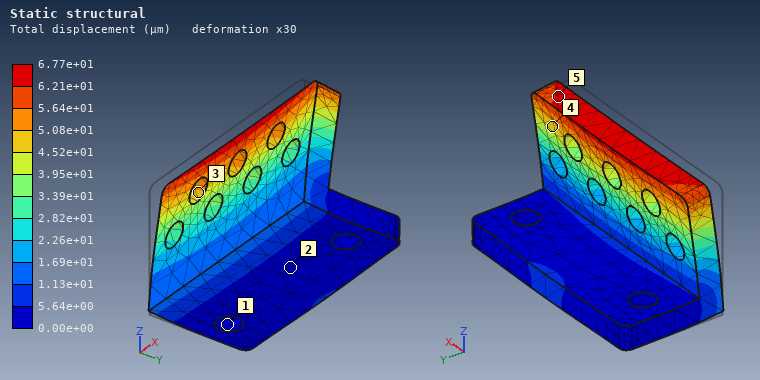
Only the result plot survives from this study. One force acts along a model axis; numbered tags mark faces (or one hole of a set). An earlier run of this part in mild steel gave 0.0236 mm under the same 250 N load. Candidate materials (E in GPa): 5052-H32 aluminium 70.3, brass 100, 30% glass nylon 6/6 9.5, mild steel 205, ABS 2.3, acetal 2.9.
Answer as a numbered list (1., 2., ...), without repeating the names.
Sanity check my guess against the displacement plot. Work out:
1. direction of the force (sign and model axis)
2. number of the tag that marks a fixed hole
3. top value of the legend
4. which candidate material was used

1. +Y
2. 1
3. 6.77e+01 µm
4. 5052-H32 aluminium
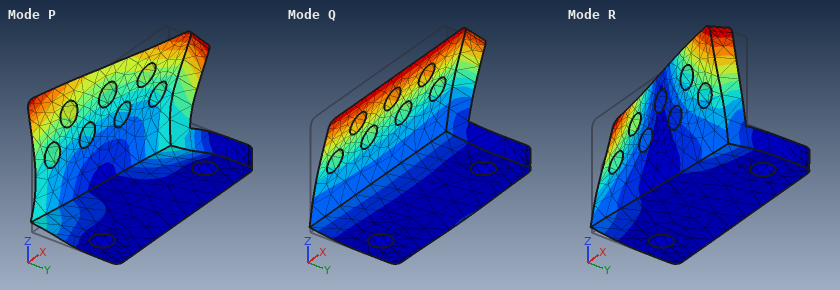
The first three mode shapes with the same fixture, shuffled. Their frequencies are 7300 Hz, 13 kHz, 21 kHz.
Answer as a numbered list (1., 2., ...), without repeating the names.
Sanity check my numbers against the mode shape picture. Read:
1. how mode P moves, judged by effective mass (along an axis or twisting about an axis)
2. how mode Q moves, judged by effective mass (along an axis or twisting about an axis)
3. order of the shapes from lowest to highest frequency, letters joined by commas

1. along X
2. along Y
3. Q, R, P
